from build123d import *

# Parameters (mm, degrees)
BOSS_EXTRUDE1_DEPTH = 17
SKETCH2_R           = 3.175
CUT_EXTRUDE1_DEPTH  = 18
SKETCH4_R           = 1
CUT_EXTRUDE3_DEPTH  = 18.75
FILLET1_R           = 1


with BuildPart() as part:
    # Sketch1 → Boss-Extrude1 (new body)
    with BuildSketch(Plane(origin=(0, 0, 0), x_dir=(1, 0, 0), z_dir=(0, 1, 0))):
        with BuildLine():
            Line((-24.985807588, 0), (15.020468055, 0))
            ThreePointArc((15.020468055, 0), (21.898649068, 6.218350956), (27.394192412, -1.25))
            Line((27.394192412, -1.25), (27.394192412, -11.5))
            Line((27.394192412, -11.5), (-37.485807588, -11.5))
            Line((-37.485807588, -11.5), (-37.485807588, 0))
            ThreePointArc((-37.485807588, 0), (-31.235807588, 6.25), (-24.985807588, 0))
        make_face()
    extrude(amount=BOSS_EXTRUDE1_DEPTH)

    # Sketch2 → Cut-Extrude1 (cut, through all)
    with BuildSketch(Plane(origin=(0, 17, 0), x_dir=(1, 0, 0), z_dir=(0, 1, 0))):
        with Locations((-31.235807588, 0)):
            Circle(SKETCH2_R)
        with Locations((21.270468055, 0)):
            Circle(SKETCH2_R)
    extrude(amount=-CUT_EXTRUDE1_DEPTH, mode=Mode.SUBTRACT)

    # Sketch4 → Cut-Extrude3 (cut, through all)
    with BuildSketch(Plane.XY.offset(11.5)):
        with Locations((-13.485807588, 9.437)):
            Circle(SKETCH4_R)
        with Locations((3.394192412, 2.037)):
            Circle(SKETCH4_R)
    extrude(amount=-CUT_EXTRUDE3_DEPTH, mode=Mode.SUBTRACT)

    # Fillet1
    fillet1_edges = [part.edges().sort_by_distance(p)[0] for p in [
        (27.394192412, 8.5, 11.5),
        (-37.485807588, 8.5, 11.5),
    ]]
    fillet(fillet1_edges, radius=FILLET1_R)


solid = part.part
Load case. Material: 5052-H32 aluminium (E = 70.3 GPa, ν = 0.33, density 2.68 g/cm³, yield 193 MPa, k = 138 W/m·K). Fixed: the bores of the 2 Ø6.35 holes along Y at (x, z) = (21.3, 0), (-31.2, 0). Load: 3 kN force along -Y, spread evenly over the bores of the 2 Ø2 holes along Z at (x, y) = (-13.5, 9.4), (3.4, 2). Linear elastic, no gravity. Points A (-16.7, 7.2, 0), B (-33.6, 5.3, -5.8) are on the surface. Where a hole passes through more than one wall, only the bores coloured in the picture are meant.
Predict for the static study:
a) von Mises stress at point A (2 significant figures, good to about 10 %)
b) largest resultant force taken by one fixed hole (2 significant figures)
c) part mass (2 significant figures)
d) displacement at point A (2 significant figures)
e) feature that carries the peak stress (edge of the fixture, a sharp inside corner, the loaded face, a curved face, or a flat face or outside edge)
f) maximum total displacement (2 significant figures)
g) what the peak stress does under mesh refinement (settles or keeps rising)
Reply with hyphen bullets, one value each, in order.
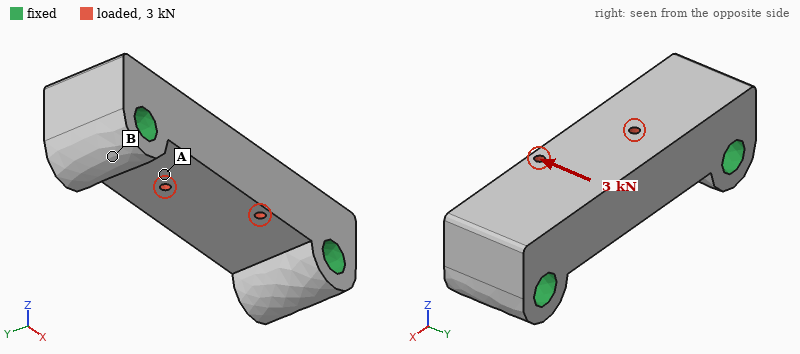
- 21 MPa
- 1.5 kN
- 36 g
- 7.8 µm
- edge of the fixture
- 12 µm
- keeps rising
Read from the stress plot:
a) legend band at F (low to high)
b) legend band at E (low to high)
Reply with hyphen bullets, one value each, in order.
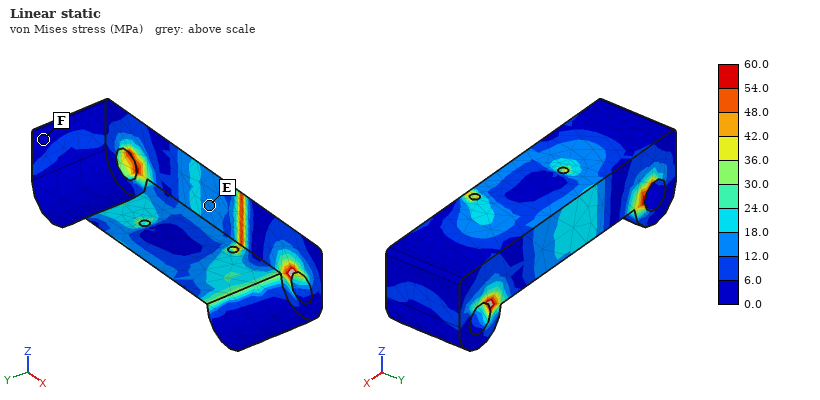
- 0.0 to 6.0 MPa
- 12.0 to 18.0 MPa
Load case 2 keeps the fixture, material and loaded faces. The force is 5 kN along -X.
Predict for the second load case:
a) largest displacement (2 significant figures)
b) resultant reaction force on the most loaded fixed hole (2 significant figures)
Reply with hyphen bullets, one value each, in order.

- 7.5 µm
- 2.5 kN
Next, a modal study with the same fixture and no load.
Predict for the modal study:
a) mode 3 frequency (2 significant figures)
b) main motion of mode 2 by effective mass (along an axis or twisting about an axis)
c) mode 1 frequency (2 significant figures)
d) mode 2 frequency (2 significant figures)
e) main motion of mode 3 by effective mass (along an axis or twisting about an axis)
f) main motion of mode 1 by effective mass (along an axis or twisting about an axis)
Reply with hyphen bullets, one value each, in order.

- 28 kHz
- along Y
- 18 kHz
- 21 kHz
- twisting about X
- along Z
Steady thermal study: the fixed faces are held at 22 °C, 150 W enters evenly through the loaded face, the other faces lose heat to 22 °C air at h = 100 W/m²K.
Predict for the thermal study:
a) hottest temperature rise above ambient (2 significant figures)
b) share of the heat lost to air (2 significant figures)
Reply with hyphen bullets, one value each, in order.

- 66 K
- 6.0 %
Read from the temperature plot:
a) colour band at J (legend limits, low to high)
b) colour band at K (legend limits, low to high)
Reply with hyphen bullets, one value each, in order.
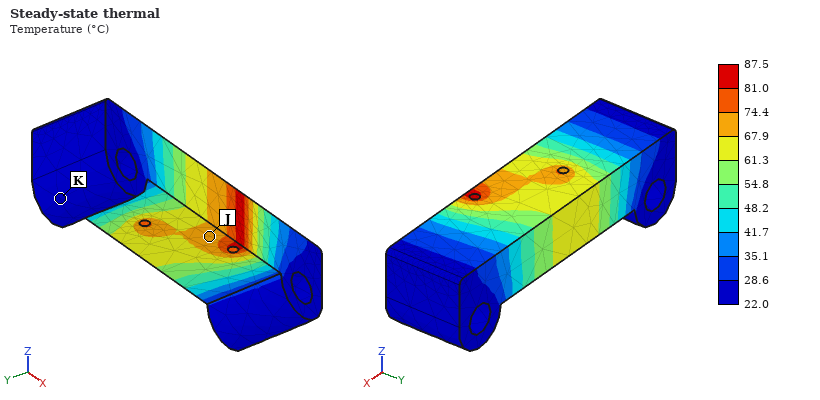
- 67.9 to 74.4 °C
- 22.0 to 28.6 °C
